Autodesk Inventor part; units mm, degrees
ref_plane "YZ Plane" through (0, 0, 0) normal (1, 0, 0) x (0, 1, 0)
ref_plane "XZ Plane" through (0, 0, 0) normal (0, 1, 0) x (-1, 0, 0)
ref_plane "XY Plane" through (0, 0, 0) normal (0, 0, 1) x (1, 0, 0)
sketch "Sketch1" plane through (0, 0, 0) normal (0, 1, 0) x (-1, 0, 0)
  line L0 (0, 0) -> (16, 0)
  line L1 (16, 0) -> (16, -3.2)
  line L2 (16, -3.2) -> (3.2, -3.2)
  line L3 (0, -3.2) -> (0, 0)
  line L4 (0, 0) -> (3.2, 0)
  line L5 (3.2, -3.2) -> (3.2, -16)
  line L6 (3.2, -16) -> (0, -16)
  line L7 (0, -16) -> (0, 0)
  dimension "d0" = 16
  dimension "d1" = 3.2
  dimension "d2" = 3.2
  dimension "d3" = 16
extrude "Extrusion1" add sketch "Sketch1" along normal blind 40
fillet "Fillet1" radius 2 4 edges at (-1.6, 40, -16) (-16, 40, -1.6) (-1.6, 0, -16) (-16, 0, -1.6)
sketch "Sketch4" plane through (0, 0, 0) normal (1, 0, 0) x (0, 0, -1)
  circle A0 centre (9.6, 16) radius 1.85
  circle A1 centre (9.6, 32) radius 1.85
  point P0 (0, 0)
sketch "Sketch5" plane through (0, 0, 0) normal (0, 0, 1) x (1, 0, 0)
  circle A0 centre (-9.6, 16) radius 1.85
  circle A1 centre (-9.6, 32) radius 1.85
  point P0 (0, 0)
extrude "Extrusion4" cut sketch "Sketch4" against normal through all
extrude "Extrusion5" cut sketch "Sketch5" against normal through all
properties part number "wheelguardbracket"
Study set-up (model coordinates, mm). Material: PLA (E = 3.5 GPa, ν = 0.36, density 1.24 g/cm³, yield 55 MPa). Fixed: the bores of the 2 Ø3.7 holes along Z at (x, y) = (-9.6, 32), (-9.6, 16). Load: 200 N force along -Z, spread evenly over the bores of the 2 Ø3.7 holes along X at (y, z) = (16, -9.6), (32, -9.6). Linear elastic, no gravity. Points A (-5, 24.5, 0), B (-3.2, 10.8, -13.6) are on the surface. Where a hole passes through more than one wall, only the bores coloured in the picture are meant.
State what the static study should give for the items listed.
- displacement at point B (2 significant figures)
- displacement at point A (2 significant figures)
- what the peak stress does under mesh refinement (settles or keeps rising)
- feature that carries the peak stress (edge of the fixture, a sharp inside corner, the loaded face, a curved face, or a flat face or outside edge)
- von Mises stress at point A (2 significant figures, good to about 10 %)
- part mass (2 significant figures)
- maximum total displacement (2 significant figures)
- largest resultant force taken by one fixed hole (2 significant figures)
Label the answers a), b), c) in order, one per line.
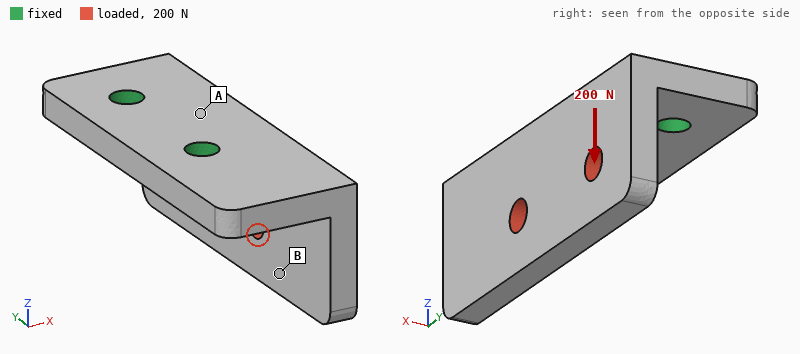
a) 0.21 mm
b) 0.057 mm
c) keeps rising
d) edge of the fixture
e) 8.1 MPa
f) 4.4 g
g) 0.30 mm
h) 100 N
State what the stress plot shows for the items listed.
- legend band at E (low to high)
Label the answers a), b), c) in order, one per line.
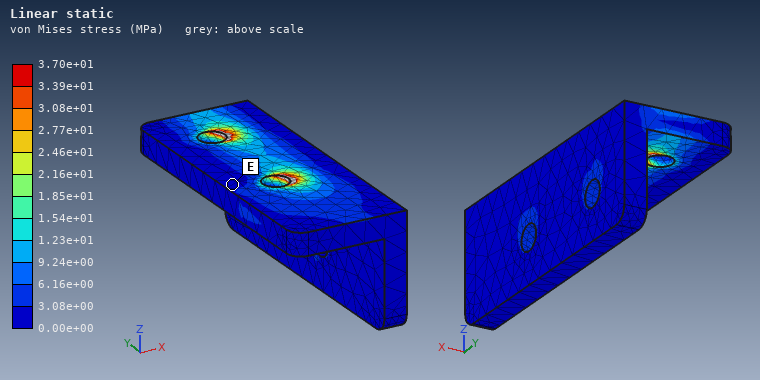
a) 0.00e+00 to 3.08e+00 MPa
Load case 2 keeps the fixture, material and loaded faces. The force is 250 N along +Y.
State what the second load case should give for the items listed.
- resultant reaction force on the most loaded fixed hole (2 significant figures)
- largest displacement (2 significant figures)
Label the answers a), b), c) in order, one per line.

a) 190 N
b) 0.27 mm
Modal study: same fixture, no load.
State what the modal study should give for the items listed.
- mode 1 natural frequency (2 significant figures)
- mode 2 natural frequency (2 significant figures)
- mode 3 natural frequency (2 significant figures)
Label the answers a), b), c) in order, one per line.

a) 2200 Hz
b) 3000 Hz
c) 4200 Hz
